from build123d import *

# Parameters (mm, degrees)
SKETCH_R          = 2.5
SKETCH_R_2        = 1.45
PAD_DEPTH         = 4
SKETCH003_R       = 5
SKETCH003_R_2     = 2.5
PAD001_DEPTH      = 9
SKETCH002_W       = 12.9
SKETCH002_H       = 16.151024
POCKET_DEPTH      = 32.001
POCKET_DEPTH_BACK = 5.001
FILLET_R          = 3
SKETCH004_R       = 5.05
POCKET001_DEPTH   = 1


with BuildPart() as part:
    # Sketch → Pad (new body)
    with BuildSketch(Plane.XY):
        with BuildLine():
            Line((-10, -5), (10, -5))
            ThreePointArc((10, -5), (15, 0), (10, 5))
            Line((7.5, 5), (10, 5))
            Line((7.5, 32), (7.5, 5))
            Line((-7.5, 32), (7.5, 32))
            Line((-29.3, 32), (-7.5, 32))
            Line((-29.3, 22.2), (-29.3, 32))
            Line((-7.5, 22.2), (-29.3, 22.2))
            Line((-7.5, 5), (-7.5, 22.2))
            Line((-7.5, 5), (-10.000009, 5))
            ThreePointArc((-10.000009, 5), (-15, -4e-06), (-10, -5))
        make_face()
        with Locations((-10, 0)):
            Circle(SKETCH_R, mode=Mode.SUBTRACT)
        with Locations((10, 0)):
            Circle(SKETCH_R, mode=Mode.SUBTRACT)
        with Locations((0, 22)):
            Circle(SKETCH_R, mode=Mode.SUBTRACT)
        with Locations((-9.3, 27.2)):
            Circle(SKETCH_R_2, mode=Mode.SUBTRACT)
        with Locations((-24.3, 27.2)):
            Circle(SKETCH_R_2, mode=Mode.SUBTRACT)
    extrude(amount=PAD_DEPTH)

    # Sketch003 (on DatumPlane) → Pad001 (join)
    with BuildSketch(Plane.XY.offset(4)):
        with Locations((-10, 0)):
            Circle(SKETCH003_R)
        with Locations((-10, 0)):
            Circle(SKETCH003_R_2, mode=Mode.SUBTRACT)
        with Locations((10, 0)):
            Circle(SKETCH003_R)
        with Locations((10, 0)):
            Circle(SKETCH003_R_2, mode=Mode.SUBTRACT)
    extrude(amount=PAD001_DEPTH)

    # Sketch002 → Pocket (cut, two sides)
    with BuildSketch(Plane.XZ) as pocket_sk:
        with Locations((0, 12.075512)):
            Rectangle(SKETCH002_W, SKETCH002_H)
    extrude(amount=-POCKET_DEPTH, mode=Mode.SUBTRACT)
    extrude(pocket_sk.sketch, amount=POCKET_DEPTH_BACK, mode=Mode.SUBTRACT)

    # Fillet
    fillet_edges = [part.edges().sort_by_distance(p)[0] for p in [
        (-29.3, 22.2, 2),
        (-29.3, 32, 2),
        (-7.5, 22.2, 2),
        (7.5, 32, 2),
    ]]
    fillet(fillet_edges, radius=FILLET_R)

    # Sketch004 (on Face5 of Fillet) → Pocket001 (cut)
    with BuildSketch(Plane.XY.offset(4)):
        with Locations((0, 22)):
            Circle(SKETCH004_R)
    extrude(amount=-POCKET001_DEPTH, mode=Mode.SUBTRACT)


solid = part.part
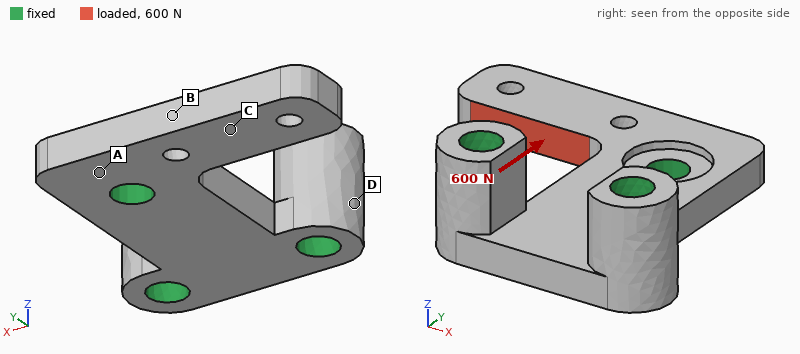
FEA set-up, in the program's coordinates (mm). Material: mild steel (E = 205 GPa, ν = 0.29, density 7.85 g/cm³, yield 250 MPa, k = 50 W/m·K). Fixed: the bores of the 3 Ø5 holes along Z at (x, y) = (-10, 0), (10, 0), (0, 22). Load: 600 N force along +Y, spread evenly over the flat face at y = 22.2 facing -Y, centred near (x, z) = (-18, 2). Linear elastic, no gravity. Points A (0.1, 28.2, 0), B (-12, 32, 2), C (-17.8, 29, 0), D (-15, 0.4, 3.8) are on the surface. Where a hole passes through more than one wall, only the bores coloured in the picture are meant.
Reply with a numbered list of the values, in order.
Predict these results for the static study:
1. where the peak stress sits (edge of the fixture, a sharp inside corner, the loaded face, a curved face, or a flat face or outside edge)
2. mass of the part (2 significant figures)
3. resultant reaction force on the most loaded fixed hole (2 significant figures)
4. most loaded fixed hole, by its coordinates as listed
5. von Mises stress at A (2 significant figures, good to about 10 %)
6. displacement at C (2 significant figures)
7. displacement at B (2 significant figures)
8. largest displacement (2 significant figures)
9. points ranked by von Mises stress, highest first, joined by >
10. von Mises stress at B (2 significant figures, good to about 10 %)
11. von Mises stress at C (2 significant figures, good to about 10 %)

1. a curved face
2. 33 g
3. 530 N
4. (0, 22)
5. 39 MPa
6. 17 µm
7. 12 µm
8. 33 µm
9. B > A > C > D
10. 56 MPa
11. 22 MPa
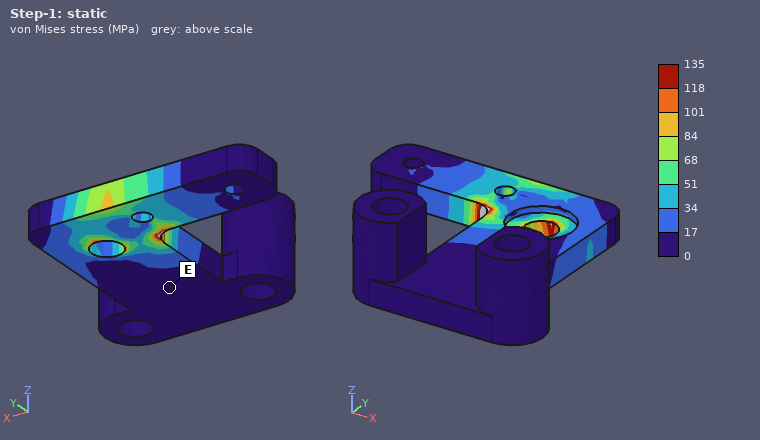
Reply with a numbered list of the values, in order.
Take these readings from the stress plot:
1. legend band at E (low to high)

1. 0 to 17 MPa
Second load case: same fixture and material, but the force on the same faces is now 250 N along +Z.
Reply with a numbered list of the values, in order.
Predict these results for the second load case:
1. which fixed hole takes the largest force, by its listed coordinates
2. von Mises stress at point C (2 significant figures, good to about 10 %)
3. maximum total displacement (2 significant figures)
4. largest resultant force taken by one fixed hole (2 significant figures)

1. (0, 22)
2. 34 MPa
3. 94 µm
4. 260 N
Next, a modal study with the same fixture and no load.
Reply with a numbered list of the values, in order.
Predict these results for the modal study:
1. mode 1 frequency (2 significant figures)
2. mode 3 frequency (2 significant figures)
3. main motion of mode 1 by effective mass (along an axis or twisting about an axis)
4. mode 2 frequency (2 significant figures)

1. 4000 Hz
2. 17 kHz
3. along Z
4. 10 kHz
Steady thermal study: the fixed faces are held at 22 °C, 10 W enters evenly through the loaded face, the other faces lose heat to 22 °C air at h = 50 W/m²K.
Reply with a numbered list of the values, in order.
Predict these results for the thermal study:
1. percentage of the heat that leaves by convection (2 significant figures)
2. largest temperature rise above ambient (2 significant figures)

1. 21 %
2. 84 K
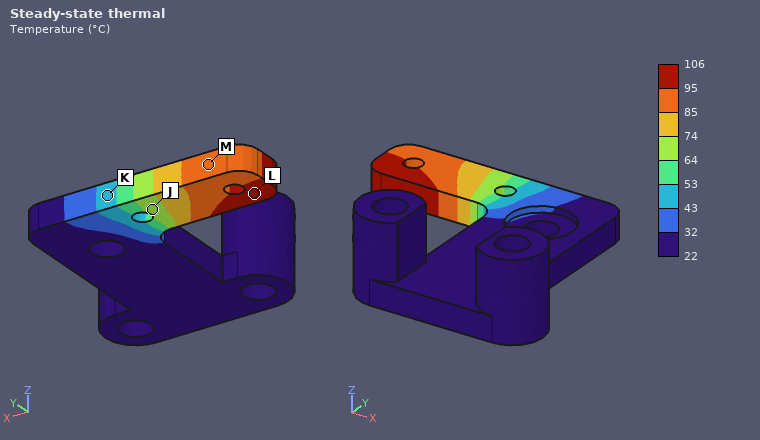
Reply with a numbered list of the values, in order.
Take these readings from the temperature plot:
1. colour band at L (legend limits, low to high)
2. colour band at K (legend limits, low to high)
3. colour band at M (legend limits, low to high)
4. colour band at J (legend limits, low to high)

1. 95 to 106 °C
2. 43 to 53 °C
3. 85 to 95 °C
4. 64 to 74 °C
